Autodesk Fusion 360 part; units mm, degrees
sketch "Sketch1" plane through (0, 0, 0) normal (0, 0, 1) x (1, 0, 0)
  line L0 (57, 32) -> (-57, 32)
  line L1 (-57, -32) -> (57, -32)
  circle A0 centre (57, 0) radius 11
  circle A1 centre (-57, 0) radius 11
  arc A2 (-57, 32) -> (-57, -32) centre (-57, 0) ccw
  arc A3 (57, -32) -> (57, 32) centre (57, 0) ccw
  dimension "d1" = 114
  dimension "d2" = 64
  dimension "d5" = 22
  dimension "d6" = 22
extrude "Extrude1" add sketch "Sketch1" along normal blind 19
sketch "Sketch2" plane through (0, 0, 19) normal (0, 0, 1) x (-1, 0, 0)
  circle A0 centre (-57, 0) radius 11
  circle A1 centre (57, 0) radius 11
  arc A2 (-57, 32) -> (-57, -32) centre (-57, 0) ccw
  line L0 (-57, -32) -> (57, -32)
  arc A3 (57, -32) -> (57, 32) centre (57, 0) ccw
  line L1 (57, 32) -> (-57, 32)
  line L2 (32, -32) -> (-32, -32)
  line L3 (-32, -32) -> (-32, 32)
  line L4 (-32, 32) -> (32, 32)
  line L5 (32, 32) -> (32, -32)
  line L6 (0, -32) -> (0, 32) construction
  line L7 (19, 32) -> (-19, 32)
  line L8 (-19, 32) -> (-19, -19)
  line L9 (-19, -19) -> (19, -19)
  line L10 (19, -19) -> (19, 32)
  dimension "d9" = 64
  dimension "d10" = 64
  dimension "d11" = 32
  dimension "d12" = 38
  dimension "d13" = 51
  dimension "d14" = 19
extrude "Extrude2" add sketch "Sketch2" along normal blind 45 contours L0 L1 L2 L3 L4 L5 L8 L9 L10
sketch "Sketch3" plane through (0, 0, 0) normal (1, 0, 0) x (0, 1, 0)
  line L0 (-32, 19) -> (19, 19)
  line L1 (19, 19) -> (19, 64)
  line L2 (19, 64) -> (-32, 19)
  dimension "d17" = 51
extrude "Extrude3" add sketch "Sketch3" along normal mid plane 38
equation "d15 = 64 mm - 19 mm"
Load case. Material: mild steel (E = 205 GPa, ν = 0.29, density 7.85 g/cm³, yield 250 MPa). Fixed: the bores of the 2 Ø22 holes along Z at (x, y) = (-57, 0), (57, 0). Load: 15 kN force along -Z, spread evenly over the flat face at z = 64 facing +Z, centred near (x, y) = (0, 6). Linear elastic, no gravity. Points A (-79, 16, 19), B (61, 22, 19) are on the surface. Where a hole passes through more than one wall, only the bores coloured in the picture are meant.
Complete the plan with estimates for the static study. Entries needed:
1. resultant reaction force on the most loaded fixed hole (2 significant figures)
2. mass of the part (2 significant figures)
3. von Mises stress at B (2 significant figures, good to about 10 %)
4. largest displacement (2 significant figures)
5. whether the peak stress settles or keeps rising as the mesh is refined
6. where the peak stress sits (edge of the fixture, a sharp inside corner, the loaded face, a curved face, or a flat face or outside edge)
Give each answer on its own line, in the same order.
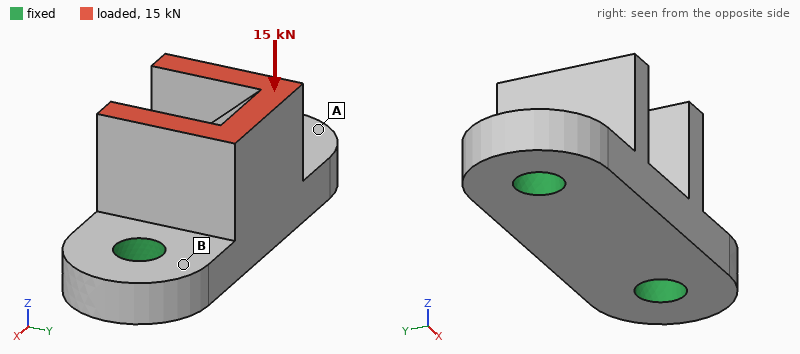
7.9 kN
2.6 kg
9.1 MPa
11 µm
keeps rising
edge of the fixture
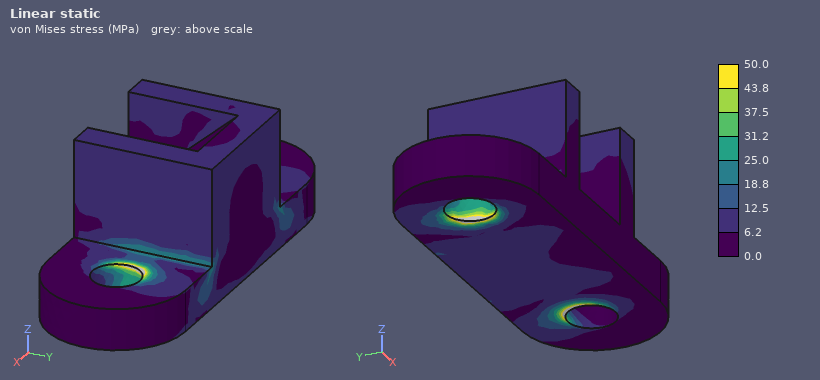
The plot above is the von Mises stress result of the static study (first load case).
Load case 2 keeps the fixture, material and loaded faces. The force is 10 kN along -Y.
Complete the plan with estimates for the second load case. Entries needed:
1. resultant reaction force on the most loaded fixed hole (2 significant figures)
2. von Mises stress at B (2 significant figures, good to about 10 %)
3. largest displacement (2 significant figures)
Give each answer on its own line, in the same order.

5.0 kN
18 MPa
40 µm
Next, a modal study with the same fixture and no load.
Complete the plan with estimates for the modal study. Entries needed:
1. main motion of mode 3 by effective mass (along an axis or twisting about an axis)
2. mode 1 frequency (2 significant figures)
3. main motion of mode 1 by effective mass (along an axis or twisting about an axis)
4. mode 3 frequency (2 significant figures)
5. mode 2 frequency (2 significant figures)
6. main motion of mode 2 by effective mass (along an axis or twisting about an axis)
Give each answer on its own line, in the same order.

along X
3600 Hz
along Y
7100 Hz
6400 Hz
along Z
